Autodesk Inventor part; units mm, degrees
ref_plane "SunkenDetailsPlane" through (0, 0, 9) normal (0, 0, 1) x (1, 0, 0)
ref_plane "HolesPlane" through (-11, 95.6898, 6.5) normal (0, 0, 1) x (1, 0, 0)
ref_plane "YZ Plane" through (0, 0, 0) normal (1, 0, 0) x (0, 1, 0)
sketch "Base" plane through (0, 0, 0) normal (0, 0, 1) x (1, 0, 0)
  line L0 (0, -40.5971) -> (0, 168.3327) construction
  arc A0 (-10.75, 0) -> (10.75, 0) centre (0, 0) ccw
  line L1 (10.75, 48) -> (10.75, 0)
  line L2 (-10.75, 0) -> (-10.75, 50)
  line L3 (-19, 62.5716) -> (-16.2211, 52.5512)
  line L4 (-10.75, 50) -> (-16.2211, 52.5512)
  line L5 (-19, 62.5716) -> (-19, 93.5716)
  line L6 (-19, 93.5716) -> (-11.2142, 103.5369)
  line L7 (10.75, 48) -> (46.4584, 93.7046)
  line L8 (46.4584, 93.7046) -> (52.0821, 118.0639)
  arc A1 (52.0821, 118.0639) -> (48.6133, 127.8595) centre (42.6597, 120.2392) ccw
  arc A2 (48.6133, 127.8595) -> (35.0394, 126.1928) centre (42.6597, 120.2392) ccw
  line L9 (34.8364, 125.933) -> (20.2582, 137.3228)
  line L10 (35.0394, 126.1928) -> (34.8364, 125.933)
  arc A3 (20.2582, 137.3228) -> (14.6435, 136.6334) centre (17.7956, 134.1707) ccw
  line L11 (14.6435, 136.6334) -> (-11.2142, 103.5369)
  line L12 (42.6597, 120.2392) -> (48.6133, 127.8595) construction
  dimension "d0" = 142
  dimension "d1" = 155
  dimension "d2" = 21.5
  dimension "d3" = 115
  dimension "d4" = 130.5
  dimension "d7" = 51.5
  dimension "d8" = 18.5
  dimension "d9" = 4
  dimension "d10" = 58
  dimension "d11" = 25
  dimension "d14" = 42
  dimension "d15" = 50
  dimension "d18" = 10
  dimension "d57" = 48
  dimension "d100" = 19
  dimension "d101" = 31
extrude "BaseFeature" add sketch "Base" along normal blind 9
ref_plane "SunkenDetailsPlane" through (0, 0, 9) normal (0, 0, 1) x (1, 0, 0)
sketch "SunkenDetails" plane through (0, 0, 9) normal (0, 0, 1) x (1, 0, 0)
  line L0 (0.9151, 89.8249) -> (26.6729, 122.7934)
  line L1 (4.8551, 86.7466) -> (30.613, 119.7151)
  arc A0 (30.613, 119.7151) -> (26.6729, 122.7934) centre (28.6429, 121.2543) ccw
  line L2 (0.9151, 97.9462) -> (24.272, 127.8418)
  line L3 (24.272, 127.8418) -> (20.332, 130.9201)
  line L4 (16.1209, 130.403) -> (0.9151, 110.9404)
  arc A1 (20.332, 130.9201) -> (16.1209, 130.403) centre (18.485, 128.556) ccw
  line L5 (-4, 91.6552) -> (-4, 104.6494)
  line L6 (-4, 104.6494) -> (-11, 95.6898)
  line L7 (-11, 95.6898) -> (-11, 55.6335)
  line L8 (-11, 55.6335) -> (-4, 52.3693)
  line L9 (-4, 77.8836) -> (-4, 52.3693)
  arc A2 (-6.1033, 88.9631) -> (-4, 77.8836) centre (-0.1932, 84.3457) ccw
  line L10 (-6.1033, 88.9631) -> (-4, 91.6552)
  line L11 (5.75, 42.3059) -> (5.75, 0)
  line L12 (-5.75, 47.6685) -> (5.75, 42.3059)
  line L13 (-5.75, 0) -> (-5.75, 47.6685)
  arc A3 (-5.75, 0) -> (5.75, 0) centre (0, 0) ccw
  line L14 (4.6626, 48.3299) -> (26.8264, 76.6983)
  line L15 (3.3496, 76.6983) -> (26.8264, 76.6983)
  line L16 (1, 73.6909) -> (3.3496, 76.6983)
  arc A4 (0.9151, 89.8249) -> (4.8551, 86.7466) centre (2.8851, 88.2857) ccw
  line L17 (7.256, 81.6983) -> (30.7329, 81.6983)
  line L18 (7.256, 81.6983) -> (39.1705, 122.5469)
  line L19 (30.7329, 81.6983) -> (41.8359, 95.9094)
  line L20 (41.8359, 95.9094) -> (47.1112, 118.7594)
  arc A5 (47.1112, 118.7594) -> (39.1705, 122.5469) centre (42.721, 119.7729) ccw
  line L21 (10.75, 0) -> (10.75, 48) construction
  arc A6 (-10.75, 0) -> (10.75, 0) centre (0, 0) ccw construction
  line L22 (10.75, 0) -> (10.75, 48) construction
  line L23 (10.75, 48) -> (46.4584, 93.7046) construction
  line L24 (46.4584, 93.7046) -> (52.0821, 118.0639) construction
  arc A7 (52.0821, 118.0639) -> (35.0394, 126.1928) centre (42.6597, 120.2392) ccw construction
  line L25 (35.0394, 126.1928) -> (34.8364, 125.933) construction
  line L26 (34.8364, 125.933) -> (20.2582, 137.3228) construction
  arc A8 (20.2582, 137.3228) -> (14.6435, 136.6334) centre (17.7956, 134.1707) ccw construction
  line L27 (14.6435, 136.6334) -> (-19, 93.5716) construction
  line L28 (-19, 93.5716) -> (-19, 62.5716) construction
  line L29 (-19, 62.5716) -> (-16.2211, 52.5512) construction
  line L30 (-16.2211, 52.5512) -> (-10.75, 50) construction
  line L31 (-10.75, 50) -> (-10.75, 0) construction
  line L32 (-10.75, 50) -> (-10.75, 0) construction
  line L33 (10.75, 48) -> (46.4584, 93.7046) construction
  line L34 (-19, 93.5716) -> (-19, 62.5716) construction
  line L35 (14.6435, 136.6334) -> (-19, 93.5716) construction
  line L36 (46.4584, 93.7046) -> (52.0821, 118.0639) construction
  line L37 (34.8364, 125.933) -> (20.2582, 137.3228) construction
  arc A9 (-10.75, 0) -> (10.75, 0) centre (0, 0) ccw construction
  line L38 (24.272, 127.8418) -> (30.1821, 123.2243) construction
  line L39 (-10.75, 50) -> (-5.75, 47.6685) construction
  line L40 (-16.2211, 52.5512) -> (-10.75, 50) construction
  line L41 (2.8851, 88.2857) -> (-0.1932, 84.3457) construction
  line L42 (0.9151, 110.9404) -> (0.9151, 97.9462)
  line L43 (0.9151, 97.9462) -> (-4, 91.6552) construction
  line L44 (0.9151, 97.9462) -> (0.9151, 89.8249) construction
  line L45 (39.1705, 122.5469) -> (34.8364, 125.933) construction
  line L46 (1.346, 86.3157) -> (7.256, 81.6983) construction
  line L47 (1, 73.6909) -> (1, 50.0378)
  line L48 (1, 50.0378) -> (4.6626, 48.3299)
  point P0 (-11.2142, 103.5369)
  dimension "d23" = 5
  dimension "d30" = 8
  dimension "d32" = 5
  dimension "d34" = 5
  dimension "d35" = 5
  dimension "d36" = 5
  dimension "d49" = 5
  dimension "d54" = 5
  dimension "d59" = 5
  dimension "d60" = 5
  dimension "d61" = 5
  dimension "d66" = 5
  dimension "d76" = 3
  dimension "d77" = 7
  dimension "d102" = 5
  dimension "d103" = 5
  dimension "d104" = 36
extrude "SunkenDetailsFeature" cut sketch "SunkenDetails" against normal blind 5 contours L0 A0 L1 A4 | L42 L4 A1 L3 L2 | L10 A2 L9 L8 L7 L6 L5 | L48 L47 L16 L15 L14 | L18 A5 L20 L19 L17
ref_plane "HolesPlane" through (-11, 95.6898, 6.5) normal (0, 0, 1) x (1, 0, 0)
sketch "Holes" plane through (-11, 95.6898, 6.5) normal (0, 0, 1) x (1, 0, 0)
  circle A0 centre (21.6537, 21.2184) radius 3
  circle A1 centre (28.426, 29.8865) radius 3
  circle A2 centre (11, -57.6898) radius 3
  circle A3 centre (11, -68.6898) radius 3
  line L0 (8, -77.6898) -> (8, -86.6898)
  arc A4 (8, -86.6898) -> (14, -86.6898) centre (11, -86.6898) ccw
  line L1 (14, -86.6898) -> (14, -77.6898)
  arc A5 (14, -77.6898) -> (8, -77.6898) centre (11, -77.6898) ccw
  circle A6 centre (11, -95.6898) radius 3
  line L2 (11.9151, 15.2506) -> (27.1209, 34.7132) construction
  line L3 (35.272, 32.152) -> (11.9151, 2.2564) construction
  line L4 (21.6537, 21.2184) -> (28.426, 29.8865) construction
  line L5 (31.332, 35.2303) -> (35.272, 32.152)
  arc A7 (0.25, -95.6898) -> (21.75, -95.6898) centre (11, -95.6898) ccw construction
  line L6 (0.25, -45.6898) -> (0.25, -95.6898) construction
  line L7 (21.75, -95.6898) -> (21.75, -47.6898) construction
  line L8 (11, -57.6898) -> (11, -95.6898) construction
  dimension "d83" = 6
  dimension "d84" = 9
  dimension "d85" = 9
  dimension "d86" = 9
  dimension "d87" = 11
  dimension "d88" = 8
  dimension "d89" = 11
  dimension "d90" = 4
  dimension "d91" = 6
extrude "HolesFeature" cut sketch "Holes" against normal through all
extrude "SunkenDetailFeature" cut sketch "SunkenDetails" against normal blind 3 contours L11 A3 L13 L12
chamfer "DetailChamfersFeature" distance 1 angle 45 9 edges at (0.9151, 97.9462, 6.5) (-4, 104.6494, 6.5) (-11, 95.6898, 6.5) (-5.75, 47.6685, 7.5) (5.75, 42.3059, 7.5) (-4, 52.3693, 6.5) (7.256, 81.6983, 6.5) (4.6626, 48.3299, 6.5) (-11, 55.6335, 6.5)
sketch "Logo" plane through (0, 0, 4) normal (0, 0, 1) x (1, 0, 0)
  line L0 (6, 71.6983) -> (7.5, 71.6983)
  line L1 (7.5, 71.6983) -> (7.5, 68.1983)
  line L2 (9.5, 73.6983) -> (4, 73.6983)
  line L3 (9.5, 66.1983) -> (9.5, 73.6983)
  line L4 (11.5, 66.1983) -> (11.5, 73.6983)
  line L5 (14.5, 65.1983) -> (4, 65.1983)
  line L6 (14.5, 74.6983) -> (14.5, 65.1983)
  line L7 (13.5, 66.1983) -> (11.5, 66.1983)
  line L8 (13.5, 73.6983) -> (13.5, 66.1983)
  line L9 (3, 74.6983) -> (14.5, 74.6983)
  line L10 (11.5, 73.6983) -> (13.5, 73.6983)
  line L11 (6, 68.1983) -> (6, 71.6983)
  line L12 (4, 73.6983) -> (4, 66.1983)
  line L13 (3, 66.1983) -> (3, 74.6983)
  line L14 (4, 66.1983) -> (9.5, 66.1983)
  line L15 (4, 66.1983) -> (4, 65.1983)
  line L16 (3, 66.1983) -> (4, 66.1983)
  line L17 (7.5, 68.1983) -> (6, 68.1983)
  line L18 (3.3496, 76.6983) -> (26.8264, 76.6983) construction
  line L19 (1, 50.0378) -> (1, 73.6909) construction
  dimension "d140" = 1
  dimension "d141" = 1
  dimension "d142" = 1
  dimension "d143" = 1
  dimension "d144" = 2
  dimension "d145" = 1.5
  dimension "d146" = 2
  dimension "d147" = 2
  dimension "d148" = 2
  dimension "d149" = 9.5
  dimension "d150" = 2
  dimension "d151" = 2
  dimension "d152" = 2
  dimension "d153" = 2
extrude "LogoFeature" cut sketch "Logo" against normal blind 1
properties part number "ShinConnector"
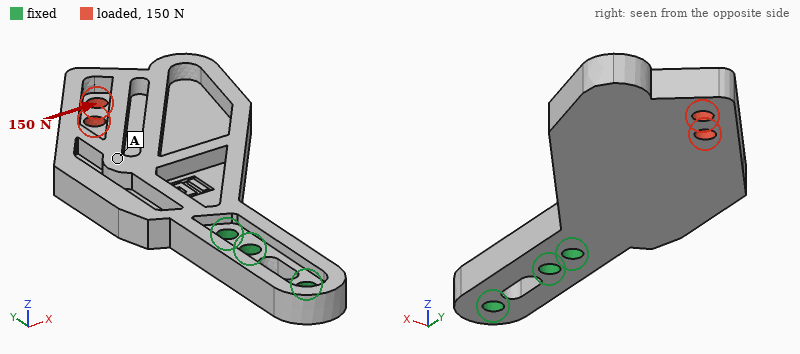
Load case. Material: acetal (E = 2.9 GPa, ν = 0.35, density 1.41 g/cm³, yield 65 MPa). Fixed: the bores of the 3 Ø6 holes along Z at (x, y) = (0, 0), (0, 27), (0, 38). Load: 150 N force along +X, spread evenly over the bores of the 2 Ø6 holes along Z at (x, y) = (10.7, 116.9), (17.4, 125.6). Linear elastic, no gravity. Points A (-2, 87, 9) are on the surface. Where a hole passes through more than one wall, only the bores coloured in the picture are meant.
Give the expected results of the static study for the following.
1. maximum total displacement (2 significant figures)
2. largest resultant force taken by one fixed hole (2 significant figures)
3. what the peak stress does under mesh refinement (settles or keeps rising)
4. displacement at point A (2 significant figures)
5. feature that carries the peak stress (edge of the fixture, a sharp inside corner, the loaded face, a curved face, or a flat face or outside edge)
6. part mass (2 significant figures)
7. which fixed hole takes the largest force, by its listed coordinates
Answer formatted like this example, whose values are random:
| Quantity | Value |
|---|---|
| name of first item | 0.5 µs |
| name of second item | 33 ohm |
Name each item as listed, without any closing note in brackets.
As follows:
| Quantity | Value |
|---|---|
| maximum total displacement | 2.0 mm |
| largest resultant force taken by one fixed hole | 600 N |
| what the peak stress does under mesh refinement | keeps rising |
| displacement at point A | 0.88 mm |
| feature that carries the peak stress | edge of the fixture |
| part mass | 50 g |
| which fixed hole takes the largest force, by its listed coordinates | (0, 38) |
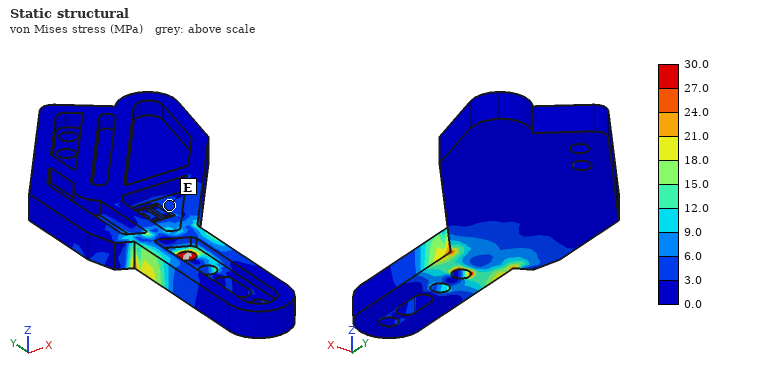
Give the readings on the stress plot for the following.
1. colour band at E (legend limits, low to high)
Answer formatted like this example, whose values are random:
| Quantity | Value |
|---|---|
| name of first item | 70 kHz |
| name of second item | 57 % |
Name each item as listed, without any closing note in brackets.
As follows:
| Quantity | Value |
|---|---|
| colour band at E | 3.0 to 6.0 MPa |
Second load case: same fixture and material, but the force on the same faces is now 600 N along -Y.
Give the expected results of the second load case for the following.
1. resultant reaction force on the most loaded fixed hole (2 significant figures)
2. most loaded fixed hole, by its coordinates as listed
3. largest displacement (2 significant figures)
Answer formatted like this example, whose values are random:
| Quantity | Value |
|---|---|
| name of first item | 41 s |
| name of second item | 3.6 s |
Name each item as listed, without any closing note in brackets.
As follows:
| Quantity | Value |
|---|---|
| resultant reaction force on the most loaded fixed hole | 580 N |
| most loaded fixed hole, by its coordinates as listed | (0, 38) |
| largest displacement | 1.9 mm |
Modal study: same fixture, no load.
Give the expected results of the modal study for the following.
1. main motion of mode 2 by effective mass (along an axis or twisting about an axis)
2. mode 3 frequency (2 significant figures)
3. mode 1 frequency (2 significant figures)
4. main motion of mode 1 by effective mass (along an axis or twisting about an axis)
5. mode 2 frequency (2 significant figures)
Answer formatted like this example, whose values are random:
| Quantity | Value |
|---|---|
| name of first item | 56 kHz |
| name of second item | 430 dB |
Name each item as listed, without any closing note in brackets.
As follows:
| Quantity | Value |
|---|---|
| main motion of mode 2 by effective mass | along X |
| mode 3 frequency | 440 Hz |
| mode 1 frequency | 150 Hz |
| main motion of mode 1 by effective mass | along Z |
| mode 2 frequency | 330 Hz |
